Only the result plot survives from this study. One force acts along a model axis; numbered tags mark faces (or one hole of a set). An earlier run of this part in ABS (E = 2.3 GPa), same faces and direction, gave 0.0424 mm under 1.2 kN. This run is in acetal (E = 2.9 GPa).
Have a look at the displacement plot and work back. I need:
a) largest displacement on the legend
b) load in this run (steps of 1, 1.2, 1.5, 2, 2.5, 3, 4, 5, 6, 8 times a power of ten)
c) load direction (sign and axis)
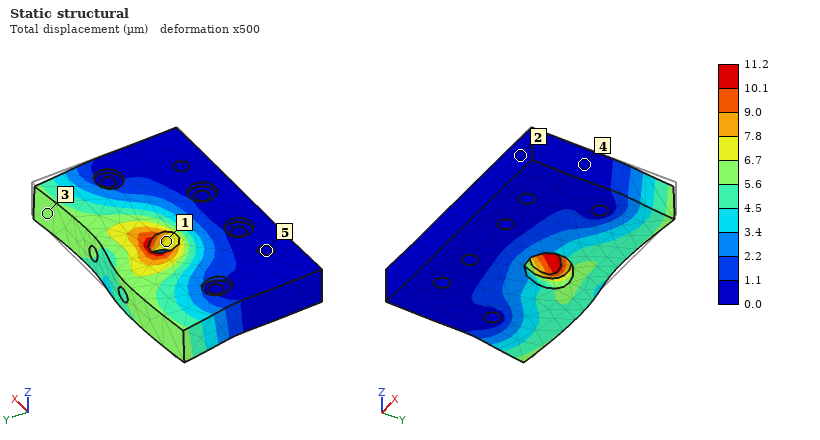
11.2 µm
400 N
-X
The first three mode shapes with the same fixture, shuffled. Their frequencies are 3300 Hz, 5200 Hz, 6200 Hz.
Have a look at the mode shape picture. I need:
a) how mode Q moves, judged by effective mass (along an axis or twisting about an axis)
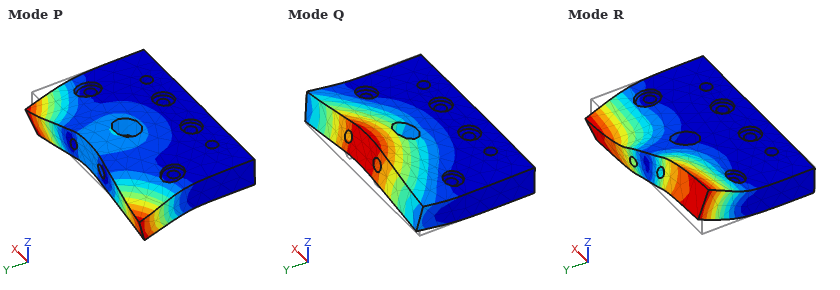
along Z
